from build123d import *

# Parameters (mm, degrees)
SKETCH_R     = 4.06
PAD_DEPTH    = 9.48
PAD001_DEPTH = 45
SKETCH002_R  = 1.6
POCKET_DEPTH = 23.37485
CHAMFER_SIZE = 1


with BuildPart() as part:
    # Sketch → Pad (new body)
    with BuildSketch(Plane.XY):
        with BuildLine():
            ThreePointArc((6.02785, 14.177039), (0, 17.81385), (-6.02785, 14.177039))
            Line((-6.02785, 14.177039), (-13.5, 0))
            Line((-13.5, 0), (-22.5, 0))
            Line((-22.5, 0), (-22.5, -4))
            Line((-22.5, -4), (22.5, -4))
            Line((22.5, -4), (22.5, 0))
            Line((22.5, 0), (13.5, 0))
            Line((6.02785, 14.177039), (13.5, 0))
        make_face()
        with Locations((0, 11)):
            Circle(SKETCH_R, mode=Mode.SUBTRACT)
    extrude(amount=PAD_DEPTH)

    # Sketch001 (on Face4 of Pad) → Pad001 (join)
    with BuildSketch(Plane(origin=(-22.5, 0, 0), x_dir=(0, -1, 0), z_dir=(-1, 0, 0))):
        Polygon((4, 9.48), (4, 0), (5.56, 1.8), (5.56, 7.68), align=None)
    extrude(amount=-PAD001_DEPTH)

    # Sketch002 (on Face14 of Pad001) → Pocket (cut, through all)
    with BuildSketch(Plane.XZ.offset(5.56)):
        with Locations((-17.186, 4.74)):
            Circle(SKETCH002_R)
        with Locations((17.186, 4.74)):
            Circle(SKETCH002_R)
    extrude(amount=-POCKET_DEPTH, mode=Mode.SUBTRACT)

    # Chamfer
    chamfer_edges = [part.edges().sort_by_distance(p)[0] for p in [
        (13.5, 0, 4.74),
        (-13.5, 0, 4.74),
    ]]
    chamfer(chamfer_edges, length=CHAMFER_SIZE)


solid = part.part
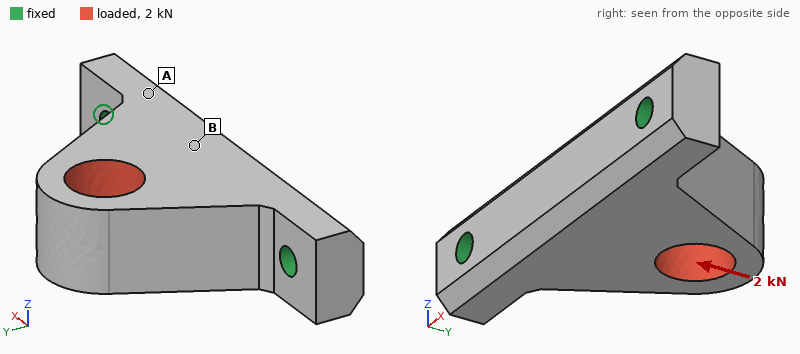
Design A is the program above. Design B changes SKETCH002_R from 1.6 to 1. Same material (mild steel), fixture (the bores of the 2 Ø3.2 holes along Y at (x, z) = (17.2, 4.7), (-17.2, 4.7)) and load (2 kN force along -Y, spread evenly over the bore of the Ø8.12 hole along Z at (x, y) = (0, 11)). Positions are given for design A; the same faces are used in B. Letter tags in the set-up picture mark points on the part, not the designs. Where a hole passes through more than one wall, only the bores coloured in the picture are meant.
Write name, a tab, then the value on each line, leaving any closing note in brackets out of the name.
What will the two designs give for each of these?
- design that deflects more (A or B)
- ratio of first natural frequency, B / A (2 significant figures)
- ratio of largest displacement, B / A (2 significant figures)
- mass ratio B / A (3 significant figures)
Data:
design that deflects more	B
ratio of first natural frequency, B / A	0.89
ratio of largest displacement, B / A	1.2
mass ratio B / A	1.01
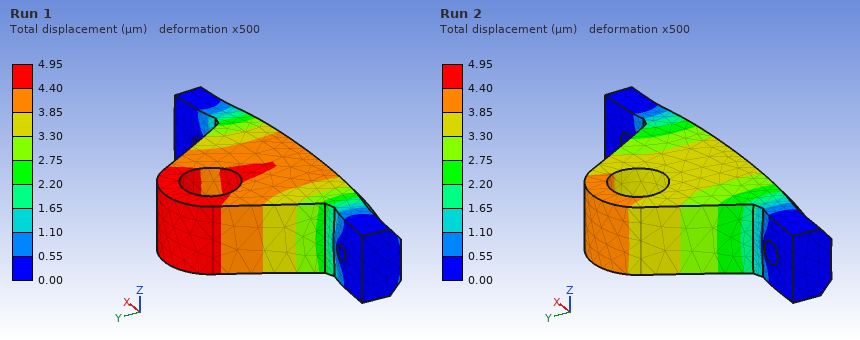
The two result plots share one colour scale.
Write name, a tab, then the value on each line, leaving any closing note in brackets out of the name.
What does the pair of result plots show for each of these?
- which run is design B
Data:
which run is design B	Run 1
